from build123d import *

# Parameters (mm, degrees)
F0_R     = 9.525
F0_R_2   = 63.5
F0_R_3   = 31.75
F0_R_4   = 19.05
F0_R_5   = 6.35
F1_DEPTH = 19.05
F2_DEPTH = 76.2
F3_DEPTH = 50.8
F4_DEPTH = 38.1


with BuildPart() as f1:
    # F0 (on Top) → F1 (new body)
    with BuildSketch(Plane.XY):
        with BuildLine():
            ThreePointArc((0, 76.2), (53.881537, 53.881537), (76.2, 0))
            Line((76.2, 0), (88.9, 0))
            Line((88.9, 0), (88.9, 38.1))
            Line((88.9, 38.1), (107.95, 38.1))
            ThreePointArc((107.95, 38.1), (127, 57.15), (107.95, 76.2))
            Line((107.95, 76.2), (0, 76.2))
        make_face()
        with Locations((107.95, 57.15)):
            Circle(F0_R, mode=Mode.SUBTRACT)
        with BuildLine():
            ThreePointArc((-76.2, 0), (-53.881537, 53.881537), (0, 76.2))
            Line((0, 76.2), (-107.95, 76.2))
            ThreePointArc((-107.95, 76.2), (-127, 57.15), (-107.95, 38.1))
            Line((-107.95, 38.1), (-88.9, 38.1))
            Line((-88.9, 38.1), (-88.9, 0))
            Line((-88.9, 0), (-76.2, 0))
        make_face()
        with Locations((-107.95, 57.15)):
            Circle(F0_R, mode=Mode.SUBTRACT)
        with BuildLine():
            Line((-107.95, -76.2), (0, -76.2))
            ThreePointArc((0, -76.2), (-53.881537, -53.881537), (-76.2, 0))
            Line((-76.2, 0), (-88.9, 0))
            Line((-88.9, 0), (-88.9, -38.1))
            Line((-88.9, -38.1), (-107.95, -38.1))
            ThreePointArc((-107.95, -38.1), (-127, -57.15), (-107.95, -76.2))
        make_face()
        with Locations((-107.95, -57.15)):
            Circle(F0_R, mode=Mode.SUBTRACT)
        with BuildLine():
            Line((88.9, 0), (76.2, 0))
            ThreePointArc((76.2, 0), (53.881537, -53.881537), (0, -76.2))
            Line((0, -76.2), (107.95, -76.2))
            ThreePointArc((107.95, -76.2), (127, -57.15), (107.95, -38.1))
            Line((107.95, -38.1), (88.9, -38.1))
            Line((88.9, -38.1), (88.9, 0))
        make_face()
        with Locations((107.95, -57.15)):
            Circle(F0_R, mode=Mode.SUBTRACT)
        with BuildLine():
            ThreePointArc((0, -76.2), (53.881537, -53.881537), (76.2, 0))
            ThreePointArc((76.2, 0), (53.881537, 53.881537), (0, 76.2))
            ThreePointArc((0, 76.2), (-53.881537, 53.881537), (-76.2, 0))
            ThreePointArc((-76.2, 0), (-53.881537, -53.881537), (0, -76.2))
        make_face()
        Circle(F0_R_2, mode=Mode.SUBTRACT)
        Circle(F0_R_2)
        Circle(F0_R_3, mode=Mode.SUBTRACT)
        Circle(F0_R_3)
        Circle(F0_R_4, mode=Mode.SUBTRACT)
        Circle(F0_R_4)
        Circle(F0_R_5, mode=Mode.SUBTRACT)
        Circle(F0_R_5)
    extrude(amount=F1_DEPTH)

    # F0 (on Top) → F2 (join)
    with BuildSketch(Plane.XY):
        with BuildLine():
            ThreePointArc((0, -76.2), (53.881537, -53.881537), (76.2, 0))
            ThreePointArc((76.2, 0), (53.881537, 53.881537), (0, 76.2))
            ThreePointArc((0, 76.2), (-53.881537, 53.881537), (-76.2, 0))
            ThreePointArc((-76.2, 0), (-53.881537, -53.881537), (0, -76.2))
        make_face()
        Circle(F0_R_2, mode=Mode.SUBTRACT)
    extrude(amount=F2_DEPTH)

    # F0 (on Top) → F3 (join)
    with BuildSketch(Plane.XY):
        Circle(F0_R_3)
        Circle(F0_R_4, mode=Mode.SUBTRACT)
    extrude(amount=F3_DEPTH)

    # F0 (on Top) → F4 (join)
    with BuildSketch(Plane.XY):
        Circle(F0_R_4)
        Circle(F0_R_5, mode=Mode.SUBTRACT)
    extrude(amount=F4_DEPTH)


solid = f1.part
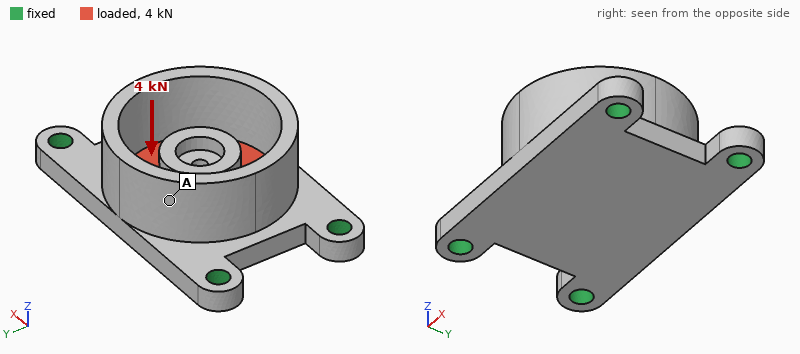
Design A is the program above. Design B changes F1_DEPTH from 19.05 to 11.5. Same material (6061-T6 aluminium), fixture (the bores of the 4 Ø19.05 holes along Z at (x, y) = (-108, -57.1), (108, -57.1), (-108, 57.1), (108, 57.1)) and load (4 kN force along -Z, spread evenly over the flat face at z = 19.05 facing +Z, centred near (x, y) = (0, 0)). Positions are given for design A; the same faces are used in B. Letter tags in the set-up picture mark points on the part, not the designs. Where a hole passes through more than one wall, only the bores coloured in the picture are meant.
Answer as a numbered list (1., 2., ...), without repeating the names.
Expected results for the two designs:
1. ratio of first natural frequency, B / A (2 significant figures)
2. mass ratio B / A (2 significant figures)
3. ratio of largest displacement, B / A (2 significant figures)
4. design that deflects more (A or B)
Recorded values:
1. 0.68
2. 0.83
3. 2.3
4. B
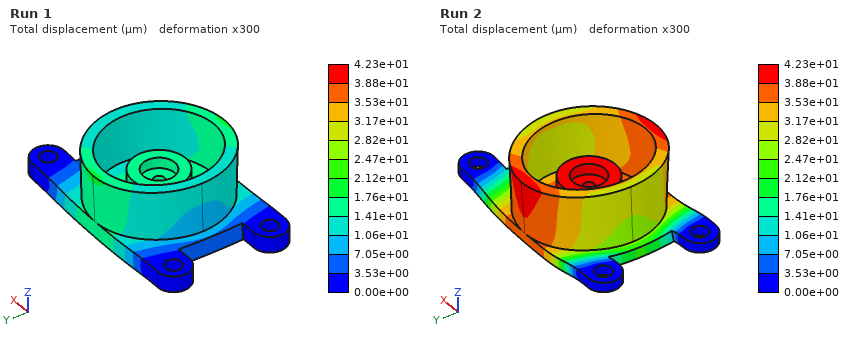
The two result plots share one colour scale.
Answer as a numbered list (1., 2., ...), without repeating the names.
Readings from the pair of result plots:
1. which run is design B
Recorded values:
1. Run 2
